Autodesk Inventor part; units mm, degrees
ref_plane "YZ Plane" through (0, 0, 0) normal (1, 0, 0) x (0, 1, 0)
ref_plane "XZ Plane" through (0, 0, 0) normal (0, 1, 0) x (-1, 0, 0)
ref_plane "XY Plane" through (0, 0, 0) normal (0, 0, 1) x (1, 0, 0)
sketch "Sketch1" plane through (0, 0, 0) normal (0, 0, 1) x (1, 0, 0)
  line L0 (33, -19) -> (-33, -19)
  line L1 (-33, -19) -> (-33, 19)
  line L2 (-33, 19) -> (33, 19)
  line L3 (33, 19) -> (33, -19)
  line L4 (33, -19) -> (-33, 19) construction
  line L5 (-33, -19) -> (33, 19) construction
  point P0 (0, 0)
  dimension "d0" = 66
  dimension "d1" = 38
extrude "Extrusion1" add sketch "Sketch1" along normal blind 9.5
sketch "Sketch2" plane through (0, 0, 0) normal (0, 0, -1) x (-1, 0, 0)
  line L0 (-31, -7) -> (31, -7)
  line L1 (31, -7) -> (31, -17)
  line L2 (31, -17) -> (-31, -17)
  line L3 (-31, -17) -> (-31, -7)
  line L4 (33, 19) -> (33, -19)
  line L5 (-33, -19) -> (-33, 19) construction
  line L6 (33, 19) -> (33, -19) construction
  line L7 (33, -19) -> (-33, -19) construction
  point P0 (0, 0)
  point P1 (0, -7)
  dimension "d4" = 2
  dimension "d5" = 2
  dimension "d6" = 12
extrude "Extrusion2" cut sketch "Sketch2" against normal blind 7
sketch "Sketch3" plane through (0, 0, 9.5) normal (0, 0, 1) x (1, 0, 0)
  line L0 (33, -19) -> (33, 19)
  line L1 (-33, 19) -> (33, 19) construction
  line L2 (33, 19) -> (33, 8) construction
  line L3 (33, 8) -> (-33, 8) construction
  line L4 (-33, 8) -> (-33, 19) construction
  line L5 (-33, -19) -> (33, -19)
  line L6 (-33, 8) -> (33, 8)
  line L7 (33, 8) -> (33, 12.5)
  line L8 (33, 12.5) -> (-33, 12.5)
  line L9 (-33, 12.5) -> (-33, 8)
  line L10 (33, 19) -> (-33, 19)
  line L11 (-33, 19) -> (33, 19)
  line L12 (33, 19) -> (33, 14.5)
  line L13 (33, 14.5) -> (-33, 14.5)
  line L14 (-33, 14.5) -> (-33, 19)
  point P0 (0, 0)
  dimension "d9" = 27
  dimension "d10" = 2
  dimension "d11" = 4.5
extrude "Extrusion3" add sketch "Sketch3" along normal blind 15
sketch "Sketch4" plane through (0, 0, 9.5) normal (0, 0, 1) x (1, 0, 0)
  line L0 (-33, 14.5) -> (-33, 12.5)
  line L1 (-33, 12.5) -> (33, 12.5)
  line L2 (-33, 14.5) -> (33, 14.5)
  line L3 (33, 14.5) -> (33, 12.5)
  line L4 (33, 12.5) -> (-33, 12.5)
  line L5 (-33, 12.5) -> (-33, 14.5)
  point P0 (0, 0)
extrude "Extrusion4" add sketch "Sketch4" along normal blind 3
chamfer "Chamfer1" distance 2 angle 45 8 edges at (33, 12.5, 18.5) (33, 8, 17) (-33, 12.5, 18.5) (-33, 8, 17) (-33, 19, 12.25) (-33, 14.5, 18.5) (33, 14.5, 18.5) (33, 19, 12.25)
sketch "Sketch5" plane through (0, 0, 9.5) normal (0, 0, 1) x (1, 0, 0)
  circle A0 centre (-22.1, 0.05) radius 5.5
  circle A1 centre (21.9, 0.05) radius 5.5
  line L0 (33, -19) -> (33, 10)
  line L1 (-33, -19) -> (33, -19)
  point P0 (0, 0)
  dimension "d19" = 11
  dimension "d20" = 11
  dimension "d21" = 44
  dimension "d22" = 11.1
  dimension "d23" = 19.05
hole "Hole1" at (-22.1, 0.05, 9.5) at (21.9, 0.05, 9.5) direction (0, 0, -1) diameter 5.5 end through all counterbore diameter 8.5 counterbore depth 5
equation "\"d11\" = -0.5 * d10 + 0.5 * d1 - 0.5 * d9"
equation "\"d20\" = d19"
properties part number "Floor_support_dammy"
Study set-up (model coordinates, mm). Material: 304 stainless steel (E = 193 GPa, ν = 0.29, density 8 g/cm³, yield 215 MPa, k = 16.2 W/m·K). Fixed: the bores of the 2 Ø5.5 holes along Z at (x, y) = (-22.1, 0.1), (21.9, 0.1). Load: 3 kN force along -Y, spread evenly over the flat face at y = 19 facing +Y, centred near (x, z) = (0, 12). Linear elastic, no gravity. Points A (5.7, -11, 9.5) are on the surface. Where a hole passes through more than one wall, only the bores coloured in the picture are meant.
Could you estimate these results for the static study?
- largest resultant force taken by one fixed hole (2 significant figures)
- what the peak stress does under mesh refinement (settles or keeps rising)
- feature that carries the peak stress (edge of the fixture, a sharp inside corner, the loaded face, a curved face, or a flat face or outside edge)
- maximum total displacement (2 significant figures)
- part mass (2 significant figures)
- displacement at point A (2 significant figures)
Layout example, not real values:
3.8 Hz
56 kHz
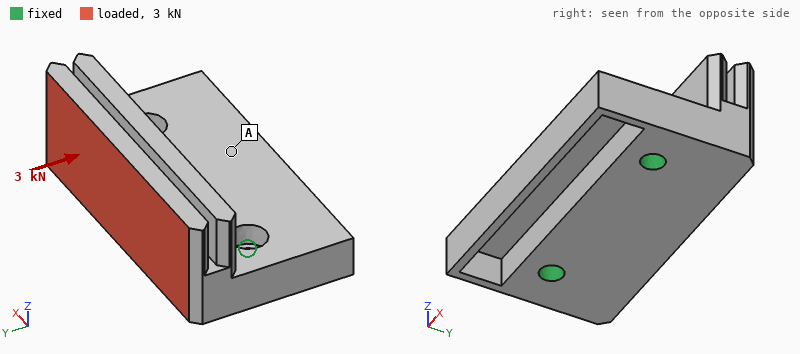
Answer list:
1.5 kN
keeps rising
edge of the fixture
36 µm
220 g
11 µm
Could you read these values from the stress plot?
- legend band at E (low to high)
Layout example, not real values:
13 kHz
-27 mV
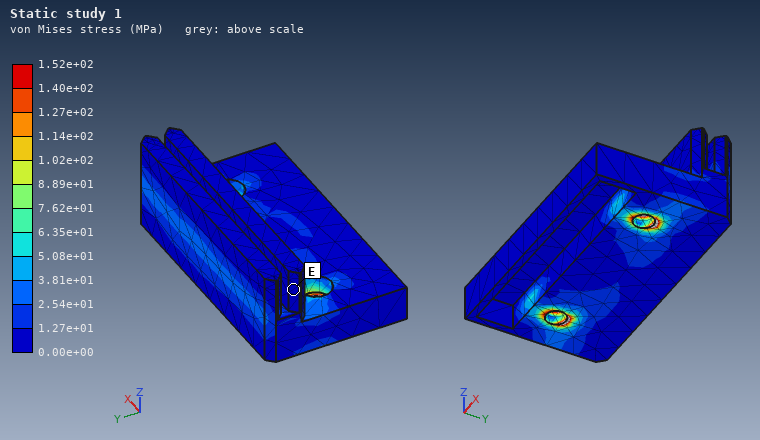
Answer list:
0.00e+00 to 1.27e+01 MPa
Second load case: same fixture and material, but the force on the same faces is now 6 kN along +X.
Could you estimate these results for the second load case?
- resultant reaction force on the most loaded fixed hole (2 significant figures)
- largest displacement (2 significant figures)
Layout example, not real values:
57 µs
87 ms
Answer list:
4.0 kN
9.8 µm
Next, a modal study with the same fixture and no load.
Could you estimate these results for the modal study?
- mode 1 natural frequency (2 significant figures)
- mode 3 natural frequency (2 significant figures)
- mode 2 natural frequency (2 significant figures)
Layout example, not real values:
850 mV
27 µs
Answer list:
4200 Hz
8400 Hz
8100 Hz
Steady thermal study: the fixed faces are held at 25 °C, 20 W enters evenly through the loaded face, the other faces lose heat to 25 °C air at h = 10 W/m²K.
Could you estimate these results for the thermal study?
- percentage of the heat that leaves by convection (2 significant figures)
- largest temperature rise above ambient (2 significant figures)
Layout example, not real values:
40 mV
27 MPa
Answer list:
15 %
64 K
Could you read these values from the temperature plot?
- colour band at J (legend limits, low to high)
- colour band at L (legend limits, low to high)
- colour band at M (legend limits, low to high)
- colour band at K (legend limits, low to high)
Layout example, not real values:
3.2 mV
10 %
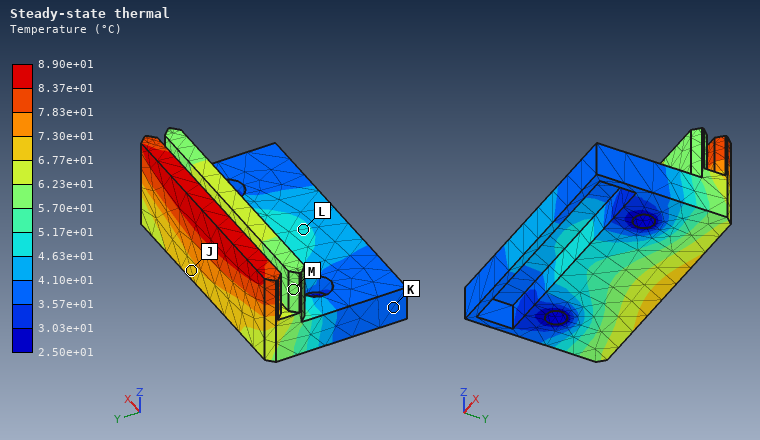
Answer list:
6.77e+01 to 7.30e+01 °C
4.63e+01 to 5.17e+01 °C
5.70e+01 to 6.23e+01 °C
3.57e+01 to 4.10e+01 °C
